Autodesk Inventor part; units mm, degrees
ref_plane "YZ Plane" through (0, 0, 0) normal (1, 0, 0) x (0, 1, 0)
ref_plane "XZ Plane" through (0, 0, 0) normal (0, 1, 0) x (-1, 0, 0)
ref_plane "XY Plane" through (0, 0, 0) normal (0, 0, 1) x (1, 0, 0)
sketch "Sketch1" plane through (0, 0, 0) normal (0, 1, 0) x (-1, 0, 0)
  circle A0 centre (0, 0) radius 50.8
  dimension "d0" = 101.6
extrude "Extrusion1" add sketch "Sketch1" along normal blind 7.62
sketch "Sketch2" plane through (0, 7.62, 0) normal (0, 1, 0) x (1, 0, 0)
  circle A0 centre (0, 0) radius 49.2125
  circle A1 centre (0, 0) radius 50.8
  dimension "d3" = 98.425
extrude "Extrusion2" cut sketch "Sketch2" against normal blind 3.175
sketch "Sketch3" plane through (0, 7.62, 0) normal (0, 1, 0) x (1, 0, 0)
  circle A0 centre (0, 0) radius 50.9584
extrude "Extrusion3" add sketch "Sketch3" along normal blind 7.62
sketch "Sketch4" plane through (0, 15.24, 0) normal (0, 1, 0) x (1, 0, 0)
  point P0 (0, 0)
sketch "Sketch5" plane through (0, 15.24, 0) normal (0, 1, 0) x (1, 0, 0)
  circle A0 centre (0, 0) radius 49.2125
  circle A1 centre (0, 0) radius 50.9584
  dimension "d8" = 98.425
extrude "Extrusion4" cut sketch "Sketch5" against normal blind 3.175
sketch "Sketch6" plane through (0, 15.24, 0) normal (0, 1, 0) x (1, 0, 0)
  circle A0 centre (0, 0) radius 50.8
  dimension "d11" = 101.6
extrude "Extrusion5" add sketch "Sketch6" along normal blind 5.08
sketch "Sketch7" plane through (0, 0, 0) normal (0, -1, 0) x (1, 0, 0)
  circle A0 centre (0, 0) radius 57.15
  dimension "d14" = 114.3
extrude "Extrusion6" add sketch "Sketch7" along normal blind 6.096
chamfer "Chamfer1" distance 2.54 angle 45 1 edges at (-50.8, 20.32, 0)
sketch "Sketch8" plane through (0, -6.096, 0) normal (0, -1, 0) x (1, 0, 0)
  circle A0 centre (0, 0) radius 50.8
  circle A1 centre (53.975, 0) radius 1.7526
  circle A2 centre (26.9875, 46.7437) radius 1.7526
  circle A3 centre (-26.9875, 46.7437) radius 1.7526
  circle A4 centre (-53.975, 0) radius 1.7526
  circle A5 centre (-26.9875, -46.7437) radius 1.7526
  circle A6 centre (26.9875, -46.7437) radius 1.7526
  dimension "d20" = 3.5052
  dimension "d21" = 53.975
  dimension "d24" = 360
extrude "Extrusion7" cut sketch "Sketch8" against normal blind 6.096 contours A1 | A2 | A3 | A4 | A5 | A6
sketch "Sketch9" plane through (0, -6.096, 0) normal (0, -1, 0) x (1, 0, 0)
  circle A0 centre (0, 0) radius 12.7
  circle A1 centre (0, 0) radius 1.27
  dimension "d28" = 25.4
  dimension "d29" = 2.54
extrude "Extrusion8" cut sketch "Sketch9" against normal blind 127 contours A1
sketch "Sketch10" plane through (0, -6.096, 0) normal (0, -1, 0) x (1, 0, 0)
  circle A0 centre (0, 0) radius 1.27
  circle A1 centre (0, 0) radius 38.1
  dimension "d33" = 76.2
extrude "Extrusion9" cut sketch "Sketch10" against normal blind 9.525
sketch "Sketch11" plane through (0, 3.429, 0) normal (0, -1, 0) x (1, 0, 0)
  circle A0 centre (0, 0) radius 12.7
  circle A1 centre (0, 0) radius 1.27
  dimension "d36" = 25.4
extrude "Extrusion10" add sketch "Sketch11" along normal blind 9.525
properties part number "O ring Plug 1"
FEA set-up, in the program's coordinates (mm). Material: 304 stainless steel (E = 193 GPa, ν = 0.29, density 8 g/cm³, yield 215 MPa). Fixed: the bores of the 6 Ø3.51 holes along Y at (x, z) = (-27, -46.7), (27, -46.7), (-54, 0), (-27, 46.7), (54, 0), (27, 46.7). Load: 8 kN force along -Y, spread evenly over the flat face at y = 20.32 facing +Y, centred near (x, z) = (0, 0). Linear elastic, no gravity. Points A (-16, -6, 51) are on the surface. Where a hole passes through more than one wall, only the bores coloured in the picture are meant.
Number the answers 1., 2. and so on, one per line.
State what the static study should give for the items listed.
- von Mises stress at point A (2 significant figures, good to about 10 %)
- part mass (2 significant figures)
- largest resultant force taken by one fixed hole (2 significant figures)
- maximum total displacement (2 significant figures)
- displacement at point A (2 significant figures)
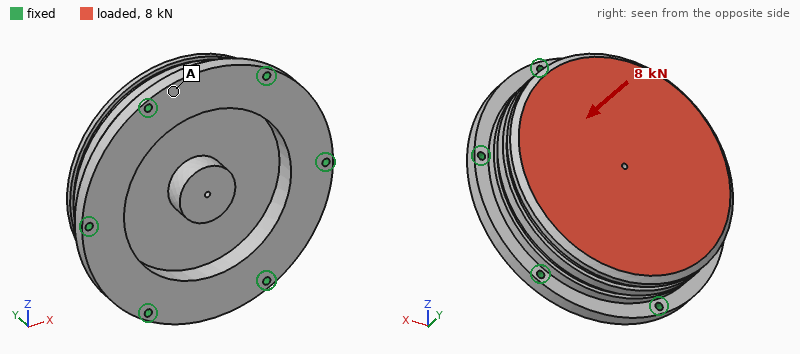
1. 7.3 MPa
2. 1.5 kg
3. 1.6 kN
4. 4.3 µm
5. 1.8 µm
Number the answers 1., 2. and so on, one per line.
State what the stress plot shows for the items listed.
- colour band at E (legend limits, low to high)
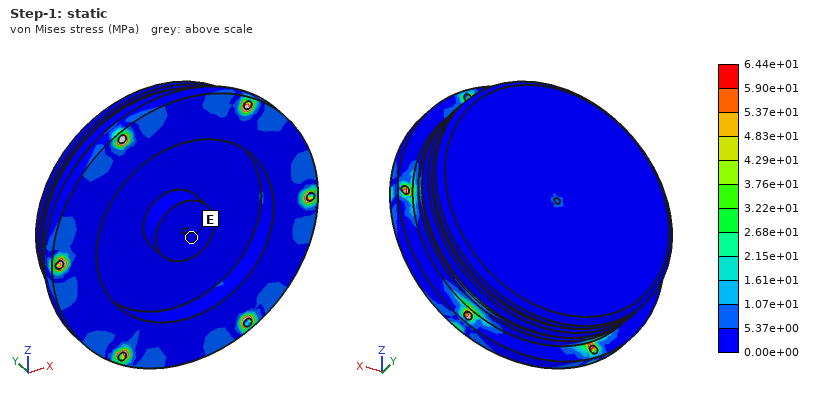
1. 0.00e+00 to 5.37e+00 MPa
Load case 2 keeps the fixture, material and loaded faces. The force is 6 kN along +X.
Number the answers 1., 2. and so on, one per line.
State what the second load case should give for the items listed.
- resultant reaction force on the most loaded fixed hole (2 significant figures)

1. 1.4 kN
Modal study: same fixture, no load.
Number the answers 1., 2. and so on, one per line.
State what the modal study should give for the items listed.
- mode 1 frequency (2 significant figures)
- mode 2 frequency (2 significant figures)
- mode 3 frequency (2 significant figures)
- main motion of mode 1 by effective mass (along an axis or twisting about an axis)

1. 7000 Hz
2. 9200 Hz
3. 9200 Hz
4. along Y
